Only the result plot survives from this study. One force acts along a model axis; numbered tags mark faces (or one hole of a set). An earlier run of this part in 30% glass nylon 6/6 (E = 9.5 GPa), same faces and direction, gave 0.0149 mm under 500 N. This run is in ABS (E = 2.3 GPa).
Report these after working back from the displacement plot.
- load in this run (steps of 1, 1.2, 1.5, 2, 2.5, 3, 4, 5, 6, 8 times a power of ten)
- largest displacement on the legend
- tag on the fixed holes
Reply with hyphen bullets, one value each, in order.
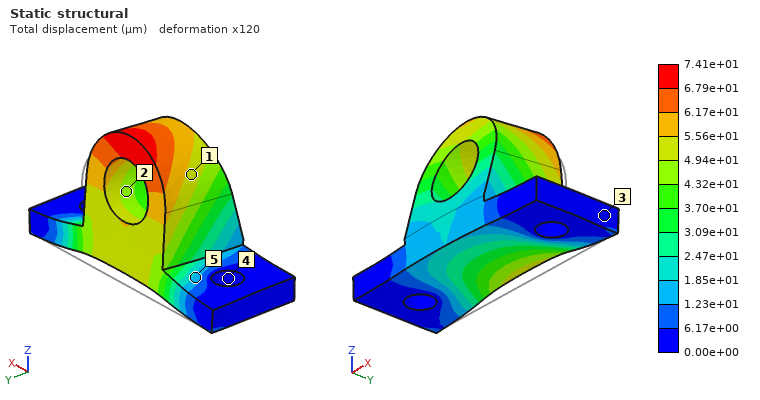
- 600 N
- 7.41e+01 µm
- 4
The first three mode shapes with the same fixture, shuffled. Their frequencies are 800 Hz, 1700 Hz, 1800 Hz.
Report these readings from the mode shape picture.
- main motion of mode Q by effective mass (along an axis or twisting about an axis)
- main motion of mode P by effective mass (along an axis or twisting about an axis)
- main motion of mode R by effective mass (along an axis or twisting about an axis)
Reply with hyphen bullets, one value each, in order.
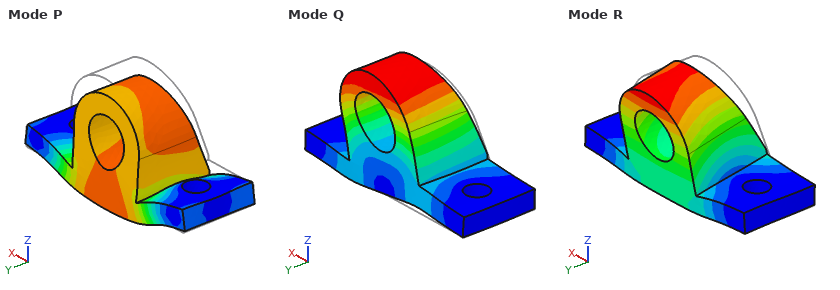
- along X
- along Z
- along Y
